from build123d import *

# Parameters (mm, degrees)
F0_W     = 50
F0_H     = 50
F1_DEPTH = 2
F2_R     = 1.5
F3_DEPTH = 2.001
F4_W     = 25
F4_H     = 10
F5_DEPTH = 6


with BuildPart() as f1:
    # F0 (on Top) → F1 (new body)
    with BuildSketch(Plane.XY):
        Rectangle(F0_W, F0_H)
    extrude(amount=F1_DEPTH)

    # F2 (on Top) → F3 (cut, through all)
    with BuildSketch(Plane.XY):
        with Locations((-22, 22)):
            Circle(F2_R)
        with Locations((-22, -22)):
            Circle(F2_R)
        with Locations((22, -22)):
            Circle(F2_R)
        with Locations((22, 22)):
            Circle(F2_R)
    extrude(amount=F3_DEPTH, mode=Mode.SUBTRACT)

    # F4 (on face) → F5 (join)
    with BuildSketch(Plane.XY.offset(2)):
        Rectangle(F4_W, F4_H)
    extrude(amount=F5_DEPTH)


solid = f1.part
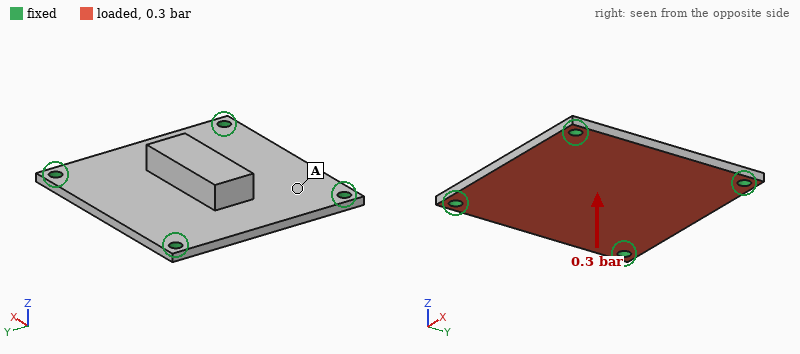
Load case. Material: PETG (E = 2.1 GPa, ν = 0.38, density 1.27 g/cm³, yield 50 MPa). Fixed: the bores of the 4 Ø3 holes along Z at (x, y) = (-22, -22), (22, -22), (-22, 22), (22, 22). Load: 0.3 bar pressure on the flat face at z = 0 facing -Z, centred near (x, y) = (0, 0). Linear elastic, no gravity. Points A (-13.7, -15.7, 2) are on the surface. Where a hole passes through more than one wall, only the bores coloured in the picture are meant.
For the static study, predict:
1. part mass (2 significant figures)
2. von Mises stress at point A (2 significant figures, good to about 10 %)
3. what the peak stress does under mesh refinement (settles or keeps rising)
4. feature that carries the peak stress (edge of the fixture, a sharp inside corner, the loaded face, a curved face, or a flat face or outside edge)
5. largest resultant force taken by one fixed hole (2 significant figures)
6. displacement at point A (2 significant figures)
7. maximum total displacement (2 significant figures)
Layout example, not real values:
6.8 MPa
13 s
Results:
8.2 g
2.2 MPa
keeps rising
edge of the fixture
19 N
0.18 mm
0.34 mm
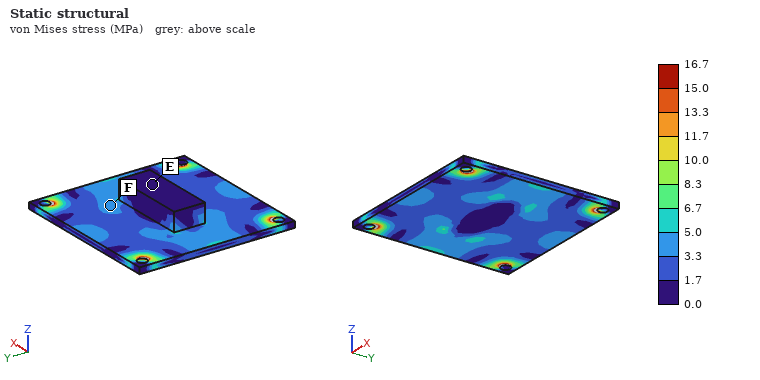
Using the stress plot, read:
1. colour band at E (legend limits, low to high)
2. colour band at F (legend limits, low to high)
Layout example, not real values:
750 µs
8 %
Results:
0.0 to 1.7 MPa
3.3 to 5.0 MPa
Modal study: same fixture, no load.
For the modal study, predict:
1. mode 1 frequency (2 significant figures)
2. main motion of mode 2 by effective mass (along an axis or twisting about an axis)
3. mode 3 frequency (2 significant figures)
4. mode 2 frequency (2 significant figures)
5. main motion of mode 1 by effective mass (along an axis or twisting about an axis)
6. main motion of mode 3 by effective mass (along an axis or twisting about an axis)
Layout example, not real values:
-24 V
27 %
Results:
820 Hz
twisting about Y
1600 Hz
1400 Hz
along Z
twisting about X
